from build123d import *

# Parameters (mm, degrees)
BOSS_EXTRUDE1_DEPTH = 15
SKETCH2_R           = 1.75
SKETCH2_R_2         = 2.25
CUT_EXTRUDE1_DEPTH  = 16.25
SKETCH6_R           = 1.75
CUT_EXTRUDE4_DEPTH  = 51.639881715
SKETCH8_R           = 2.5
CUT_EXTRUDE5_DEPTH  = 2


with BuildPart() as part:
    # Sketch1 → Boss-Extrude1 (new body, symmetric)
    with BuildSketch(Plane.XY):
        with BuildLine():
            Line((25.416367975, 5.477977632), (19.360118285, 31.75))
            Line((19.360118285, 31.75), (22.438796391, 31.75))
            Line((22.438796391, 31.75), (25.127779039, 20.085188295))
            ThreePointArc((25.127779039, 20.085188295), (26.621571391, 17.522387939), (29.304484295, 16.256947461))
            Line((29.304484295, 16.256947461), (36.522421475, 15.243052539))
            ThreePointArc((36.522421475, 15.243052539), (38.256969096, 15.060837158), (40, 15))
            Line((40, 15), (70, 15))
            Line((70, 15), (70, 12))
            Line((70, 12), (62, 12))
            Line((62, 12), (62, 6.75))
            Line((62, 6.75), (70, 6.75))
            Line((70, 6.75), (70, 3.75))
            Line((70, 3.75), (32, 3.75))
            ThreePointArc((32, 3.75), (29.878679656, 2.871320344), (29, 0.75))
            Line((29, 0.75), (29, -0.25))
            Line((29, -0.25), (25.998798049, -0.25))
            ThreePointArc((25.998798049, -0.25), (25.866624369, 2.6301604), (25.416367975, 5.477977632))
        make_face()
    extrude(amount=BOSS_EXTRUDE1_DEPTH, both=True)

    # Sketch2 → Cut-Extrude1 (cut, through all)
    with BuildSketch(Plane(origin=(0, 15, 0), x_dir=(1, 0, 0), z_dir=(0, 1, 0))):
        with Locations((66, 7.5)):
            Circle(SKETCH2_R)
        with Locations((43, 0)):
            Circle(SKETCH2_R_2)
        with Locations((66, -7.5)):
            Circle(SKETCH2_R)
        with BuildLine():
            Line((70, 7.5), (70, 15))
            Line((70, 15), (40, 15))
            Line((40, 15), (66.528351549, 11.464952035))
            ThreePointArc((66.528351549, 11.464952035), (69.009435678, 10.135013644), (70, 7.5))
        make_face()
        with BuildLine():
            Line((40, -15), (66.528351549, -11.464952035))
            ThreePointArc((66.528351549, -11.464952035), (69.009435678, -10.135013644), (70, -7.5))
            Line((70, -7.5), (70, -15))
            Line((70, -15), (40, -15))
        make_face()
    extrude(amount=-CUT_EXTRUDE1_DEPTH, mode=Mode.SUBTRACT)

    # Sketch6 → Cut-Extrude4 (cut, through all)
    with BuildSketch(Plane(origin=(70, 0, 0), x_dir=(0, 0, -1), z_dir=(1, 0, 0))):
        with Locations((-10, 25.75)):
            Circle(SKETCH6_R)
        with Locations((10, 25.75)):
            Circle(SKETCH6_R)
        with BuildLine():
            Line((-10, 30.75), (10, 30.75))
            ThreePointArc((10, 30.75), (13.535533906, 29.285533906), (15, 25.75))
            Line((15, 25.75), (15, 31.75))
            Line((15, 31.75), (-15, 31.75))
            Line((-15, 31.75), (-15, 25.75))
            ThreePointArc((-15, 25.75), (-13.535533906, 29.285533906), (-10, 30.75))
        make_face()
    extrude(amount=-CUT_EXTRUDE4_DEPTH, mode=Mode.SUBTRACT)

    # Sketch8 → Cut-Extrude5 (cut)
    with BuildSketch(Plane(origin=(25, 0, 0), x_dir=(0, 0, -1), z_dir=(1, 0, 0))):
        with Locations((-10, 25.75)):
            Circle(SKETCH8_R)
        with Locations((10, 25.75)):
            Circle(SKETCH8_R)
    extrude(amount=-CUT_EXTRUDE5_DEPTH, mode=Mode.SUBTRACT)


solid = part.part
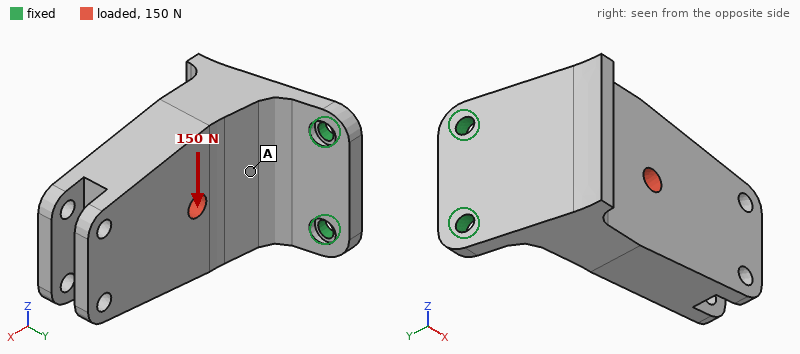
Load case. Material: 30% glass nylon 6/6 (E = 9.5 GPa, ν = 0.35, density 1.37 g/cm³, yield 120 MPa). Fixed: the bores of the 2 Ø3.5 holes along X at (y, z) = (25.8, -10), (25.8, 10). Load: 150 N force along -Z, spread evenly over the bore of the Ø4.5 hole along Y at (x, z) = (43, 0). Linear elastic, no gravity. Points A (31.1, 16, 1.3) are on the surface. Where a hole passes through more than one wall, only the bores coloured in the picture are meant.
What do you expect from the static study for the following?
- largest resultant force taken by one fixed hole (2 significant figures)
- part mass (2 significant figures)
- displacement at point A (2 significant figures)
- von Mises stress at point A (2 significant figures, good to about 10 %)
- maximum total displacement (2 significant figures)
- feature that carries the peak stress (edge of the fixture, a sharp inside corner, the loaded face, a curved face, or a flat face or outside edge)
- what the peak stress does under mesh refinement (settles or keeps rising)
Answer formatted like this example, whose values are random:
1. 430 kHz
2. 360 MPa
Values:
1. 200 N
2. 20 g
3. 0.043 mm
4. 4.9 MPa
5. 0.26 mm
6. edge of the fixture
7. keeps rising
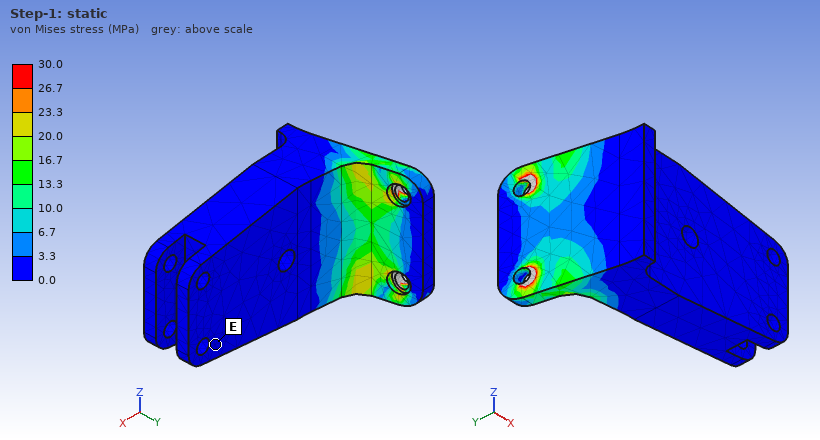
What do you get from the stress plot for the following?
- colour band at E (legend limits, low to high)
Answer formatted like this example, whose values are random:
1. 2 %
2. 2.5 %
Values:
1. 0.0 to 3.3 MPa
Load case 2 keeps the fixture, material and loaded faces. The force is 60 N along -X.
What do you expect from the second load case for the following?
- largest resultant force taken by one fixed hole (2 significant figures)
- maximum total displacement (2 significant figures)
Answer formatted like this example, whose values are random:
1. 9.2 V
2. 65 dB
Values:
1. 30 N
2. 0.66 mm
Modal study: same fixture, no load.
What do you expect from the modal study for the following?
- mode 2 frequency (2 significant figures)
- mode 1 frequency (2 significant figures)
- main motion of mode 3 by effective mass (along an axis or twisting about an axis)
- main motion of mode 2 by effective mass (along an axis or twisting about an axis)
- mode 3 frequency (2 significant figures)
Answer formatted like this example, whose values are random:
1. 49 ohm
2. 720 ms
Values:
1. 1100 Hz
2. 320 Hz
3. along X
4. along Z
5. 2900 Hz
